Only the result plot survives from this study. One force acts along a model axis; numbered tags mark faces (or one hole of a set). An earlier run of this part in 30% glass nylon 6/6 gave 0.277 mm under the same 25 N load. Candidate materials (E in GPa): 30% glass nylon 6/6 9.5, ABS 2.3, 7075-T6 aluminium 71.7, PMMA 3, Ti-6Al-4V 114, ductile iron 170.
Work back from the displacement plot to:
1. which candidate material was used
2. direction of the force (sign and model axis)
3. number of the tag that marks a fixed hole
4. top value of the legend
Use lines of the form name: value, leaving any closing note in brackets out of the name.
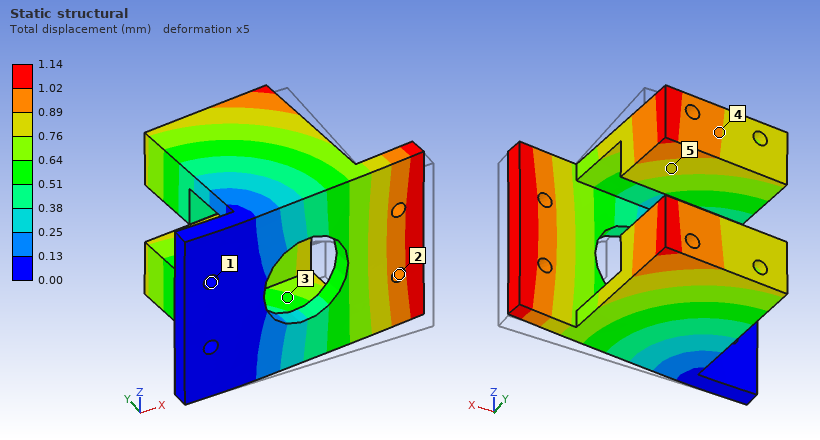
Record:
which candidate material was used: ABS
direction of the force: +Y
number of the tag that marks a fixed hole: 1
top value of the legend: 1.14 mm
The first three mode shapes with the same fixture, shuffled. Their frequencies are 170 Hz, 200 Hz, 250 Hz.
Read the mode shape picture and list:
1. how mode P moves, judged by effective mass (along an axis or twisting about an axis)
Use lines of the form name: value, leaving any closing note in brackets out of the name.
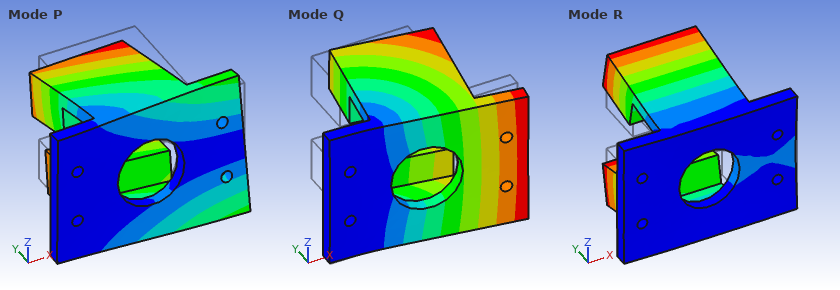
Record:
how mode P moves, judged by effective mass: along Z
